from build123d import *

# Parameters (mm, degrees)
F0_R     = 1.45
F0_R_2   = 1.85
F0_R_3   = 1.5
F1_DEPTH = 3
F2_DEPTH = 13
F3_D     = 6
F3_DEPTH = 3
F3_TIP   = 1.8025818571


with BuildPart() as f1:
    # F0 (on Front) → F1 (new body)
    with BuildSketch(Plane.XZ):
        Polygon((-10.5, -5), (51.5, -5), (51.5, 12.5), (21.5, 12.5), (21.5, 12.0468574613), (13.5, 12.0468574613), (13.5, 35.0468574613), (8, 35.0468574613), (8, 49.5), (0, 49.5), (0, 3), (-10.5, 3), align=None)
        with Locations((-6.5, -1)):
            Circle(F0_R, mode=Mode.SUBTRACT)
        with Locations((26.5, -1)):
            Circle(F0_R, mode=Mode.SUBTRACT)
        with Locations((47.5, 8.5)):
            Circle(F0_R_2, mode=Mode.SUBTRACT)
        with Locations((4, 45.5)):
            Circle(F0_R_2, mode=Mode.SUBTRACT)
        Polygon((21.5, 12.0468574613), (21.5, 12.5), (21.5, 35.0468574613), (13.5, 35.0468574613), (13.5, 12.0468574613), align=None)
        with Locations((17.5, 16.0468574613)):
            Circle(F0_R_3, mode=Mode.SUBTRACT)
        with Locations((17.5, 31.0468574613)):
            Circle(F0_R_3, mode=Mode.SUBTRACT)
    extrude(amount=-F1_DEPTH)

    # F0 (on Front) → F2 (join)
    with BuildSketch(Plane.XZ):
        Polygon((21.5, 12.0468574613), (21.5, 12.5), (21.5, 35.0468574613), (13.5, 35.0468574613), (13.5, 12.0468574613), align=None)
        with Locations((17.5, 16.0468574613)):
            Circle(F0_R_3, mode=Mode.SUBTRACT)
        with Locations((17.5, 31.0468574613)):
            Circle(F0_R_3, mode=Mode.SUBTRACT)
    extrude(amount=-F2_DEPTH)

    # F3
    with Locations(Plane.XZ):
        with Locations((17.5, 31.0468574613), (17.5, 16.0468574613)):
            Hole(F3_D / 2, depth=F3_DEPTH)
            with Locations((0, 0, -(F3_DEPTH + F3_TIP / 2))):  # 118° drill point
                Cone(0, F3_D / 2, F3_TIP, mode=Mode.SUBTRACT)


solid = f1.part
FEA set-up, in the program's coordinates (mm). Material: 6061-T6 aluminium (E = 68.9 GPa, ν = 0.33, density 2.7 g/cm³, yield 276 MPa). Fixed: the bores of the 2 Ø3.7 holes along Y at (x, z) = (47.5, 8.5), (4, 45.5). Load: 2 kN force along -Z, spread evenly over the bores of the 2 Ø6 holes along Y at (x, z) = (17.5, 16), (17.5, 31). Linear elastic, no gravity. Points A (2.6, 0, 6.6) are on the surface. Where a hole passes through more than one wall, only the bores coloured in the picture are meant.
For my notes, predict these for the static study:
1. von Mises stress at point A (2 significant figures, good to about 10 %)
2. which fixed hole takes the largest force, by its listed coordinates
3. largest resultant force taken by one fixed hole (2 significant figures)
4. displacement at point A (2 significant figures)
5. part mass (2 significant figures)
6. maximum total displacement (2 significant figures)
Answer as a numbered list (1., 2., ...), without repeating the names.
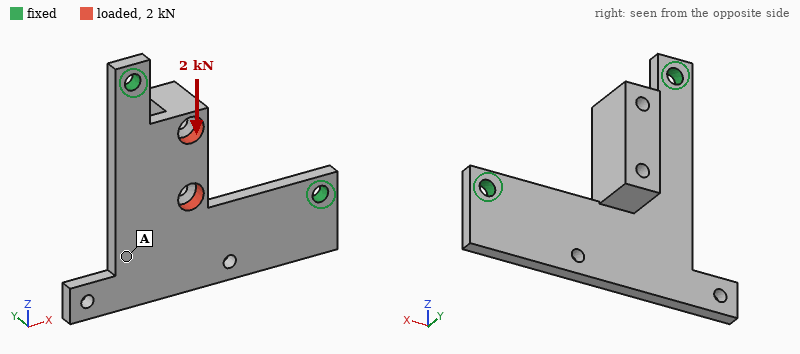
1. 19 MPa
2. (4, 45.5)
3. 1.7 kN
4. 23 µm
5. 17 g
6. 49 µm
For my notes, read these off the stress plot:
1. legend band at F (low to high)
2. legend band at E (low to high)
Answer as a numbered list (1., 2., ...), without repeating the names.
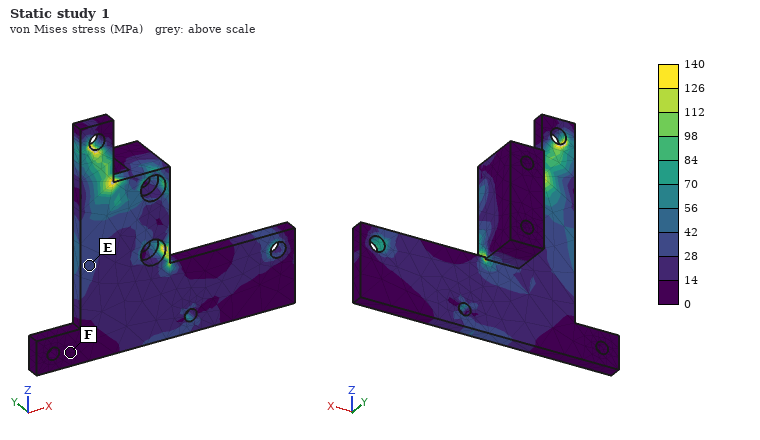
1. 0 to 14 MPa
2. 28 to 42 MPa
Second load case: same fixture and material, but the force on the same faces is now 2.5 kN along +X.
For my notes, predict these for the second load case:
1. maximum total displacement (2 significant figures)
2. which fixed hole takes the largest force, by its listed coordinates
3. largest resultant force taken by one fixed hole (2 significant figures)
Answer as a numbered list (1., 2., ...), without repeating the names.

1. 71 µm
2. (47.5, 8.5)
3. 1.5 kN
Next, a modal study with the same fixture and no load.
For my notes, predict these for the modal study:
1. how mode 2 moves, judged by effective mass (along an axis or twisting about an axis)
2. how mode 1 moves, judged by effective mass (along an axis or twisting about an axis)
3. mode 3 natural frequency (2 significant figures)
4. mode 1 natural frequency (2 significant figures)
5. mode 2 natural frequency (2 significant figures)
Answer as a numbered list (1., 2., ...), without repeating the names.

1. along Y
2. along Y
3. 5500 Hz
4. 1200 Hz
5. 3200 Hz
